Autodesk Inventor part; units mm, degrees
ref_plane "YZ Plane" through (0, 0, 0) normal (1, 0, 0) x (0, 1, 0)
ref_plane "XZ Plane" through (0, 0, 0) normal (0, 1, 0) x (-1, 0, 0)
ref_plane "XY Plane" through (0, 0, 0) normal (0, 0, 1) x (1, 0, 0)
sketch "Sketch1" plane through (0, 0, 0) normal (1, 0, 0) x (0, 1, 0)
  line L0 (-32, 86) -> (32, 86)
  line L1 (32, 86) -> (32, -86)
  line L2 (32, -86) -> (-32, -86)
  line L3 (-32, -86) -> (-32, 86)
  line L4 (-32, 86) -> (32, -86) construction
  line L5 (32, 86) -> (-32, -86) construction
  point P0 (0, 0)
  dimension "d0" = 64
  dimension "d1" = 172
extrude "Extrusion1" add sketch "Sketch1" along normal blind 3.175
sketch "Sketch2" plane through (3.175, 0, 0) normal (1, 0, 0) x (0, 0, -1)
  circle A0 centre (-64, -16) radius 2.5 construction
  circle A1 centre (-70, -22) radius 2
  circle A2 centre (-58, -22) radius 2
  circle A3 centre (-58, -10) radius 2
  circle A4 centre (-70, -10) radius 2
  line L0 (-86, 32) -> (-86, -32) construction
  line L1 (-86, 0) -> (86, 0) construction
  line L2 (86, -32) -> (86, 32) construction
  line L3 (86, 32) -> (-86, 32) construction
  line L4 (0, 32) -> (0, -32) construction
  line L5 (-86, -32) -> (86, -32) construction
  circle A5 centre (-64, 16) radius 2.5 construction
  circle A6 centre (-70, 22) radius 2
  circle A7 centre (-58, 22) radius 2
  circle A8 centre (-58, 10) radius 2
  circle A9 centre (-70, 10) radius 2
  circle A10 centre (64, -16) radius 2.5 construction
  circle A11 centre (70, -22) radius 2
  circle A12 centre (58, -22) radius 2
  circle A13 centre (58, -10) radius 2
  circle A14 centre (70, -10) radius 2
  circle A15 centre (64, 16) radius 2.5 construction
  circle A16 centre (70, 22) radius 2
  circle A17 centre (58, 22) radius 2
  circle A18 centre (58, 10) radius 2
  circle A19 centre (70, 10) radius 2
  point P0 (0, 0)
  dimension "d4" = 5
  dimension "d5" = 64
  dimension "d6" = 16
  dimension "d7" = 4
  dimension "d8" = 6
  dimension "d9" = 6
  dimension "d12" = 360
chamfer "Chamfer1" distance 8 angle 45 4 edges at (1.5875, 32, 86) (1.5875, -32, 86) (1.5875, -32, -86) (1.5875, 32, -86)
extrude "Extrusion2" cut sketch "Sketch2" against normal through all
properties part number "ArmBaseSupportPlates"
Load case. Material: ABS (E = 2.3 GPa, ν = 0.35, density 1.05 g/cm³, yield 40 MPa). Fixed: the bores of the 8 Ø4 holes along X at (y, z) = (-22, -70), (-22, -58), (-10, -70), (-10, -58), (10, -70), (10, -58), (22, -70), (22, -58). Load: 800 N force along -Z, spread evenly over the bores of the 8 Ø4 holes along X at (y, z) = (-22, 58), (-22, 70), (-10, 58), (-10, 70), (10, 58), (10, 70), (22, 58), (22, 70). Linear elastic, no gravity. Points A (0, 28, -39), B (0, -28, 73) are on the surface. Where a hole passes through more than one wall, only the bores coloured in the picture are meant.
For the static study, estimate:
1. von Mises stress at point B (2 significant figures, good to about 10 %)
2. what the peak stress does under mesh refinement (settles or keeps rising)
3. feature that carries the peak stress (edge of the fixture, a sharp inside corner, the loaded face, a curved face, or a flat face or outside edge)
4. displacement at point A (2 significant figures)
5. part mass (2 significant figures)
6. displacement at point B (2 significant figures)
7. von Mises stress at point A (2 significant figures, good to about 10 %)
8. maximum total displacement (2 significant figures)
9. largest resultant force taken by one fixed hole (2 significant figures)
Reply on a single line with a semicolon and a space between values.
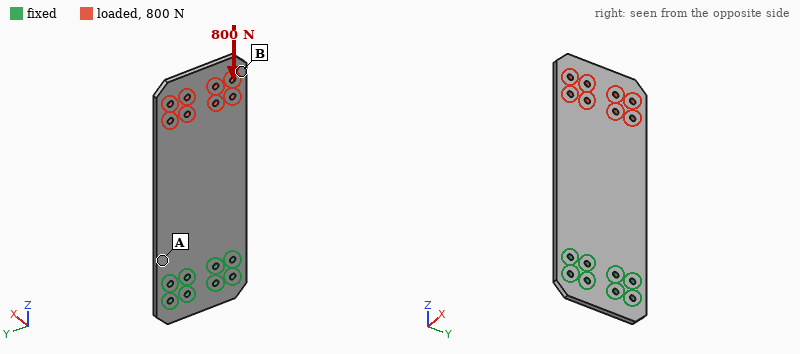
1.1 MPa; keeps rising; edge of the fixture; 0.041 mm; 36 g; 0.21 mm; 3.6 MPa; 0.22 mm; 180 N
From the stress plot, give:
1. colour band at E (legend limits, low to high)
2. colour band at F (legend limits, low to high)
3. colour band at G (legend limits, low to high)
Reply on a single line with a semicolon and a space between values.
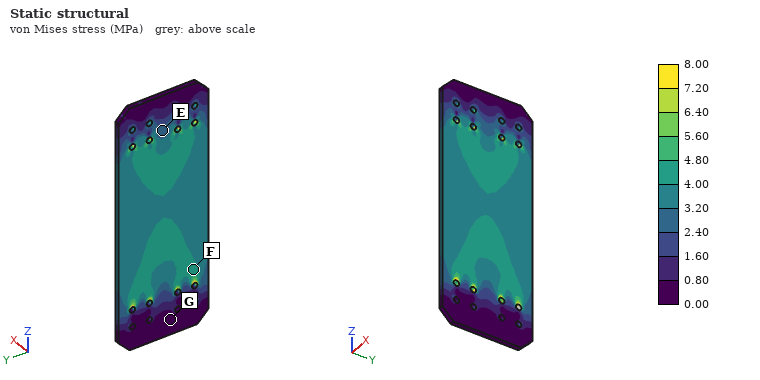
2.40 to 3.20 MPa; 4.00 to 4.80 MPa; 0.00 to 0.80 MPa
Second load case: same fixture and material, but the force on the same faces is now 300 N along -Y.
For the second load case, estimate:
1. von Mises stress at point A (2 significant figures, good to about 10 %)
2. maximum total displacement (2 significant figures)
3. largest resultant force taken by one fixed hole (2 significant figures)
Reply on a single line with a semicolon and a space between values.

12 MPa; 1.8 mm; 550 N
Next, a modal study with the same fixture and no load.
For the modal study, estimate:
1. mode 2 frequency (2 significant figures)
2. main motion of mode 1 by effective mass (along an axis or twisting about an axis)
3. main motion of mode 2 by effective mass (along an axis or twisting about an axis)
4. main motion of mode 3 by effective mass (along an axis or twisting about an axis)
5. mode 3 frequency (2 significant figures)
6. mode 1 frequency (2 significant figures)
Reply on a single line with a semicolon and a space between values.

180 Hz; along X; twisting about Z; along X; 240 Hz; 39 Hz
